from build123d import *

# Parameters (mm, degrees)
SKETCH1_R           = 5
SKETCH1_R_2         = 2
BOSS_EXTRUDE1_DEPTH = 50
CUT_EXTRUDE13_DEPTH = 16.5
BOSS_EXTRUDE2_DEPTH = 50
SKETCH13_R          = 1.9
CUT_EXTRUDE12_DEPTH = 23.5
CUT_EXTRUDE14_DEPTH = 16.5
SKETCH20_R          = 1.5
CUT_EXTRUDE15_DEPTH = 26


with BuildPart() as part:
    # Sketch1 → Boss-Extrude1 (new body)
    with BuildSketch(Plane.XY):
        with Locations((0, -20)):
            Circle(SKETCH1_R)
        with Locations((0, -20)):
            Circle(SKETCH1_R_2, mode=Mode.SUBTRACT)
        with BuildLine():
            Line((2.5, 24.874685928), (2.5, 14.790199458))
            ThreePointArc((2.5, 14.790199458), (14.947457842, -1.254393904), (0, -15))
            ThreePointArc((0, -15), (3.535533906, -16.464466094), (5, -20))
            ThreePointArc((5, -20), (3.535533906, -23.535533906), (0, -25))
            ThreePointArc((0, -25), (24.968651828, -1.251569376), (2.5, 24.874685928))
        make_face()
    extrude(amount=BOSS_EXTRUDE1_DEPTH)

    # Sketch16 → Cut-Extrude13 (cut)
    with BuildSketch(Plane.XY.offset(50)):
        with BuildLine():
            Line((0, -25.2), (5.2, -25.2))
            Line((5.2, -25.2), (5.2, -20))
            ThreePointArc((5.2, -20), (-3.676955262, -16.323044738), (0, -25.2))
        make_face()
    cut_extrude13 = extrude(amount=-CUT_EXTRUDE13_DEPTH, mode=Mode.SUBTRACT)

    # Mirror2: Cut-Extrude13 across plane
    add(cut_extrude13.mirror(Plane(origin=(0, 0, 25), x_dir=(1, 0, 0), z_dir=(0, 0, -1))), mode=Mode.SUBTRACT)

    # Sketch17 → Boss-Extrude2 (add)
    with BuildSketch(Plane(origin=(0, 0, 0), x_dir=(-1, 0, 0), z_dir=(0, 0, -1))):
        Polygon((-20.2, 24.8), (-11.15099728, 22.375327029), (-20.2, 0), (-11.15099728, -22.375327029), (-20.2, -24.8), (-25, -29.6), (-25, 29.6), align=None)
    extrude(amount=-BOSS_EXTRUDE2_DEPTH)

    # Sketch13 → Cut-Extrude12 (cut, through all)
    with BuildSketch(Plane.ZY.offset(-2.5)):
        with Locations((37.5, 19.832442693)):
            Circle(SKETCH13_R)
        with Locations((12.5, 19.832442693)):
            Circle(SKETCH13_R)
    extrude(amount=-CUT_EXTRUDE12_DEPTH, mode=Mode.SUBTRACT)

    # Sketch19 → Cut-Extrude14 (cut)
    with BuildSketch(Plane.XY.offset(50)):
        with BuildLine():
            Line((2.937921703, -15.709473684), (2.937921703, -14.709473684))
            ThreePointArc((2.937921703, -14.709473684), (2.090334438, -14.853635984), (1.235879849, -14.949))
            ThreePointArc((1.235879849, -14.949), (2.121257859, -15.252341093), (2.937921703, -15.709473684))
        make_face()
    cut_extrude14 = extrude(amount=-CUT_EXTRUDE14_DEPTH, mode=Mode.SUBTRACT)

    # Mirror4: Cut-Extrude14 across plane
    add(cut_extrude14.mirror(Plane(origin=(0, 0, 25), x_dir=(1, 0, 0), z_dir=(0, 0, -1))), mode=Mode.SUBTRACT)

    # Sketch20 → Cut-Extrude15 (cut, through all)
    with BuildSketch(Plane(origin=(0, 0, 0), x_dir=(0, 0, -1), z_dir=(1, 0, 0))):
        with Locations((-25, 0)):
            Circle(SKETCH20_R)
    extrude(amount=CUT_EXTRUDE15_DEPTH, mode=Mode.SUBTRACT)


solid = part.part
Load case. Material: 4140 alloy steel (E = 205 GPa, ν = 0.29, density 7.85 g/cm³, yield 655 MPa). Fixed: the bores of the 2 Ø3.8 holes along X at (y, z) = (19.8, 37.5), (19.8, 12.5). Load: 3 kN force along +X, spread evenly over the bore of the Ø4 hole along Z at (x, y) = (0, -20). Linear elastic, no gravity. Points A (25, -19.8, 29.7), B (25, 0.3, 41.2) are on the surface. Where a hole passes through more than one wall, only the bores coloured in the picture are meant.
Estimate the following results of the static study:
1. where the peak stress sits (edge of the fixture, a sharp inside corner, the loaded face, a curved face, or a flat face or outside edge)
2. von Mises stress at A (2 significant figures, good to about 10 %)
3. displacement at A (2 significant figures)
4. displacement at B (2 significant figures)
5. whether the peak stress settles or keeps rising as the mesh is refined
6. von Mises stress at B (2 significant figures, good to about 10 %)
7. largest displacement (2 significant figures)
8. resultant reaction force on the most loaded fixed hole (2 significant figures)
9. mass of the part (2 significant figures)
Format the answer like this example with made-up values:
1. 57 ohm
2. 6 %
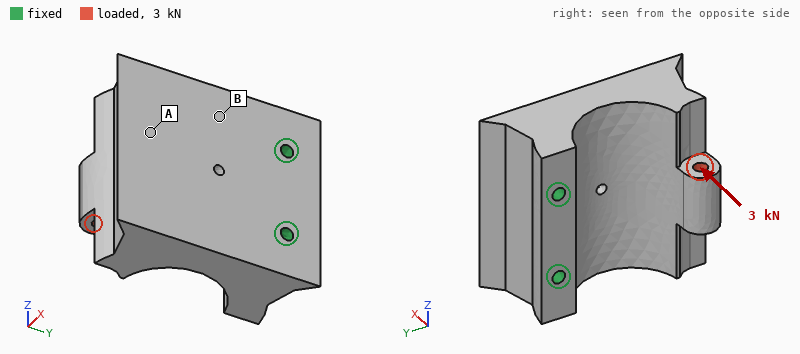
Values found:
1. a sharp inside corner
2. 11 MPa
3. 42 µm
4. 12 µm
5. keeps rising
6. 66 MPa
7. 62 µm
8. 1.5 kN
9. 320 g
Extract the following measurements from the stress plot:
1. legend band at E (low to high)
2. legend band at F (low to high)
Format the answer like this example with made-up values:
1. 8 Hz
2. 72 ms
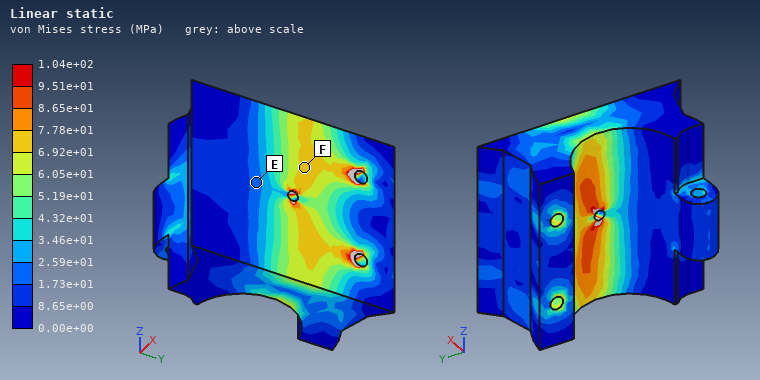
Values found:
1. 1.73e+01 to 2.59e+01 MPa
2. 6.92e+01 to 7.78e+01 MPa
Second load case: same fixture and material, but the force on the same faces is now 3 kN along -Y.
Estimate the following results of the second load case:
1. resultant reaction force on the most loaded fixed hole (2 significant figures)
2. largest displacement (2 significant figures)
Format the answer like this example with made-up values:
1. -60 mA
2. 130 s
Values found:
1. 1.5 kN
2. 61 µm
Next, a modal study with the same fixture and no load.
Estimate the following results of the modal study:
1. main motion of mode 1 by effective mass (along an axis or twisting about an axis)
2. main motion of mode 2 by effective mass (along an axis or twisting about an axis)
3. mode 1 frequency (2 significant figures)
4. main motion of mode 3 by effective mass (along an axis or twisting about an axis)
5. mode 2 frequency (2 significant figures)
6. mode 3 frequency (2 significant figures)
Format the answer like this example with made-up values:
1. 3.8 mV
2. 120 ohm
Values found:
1. along X
2. along Z
3. 3900 Hz
4. along Z
5. 7200 Hz
6. 9400 Hz
